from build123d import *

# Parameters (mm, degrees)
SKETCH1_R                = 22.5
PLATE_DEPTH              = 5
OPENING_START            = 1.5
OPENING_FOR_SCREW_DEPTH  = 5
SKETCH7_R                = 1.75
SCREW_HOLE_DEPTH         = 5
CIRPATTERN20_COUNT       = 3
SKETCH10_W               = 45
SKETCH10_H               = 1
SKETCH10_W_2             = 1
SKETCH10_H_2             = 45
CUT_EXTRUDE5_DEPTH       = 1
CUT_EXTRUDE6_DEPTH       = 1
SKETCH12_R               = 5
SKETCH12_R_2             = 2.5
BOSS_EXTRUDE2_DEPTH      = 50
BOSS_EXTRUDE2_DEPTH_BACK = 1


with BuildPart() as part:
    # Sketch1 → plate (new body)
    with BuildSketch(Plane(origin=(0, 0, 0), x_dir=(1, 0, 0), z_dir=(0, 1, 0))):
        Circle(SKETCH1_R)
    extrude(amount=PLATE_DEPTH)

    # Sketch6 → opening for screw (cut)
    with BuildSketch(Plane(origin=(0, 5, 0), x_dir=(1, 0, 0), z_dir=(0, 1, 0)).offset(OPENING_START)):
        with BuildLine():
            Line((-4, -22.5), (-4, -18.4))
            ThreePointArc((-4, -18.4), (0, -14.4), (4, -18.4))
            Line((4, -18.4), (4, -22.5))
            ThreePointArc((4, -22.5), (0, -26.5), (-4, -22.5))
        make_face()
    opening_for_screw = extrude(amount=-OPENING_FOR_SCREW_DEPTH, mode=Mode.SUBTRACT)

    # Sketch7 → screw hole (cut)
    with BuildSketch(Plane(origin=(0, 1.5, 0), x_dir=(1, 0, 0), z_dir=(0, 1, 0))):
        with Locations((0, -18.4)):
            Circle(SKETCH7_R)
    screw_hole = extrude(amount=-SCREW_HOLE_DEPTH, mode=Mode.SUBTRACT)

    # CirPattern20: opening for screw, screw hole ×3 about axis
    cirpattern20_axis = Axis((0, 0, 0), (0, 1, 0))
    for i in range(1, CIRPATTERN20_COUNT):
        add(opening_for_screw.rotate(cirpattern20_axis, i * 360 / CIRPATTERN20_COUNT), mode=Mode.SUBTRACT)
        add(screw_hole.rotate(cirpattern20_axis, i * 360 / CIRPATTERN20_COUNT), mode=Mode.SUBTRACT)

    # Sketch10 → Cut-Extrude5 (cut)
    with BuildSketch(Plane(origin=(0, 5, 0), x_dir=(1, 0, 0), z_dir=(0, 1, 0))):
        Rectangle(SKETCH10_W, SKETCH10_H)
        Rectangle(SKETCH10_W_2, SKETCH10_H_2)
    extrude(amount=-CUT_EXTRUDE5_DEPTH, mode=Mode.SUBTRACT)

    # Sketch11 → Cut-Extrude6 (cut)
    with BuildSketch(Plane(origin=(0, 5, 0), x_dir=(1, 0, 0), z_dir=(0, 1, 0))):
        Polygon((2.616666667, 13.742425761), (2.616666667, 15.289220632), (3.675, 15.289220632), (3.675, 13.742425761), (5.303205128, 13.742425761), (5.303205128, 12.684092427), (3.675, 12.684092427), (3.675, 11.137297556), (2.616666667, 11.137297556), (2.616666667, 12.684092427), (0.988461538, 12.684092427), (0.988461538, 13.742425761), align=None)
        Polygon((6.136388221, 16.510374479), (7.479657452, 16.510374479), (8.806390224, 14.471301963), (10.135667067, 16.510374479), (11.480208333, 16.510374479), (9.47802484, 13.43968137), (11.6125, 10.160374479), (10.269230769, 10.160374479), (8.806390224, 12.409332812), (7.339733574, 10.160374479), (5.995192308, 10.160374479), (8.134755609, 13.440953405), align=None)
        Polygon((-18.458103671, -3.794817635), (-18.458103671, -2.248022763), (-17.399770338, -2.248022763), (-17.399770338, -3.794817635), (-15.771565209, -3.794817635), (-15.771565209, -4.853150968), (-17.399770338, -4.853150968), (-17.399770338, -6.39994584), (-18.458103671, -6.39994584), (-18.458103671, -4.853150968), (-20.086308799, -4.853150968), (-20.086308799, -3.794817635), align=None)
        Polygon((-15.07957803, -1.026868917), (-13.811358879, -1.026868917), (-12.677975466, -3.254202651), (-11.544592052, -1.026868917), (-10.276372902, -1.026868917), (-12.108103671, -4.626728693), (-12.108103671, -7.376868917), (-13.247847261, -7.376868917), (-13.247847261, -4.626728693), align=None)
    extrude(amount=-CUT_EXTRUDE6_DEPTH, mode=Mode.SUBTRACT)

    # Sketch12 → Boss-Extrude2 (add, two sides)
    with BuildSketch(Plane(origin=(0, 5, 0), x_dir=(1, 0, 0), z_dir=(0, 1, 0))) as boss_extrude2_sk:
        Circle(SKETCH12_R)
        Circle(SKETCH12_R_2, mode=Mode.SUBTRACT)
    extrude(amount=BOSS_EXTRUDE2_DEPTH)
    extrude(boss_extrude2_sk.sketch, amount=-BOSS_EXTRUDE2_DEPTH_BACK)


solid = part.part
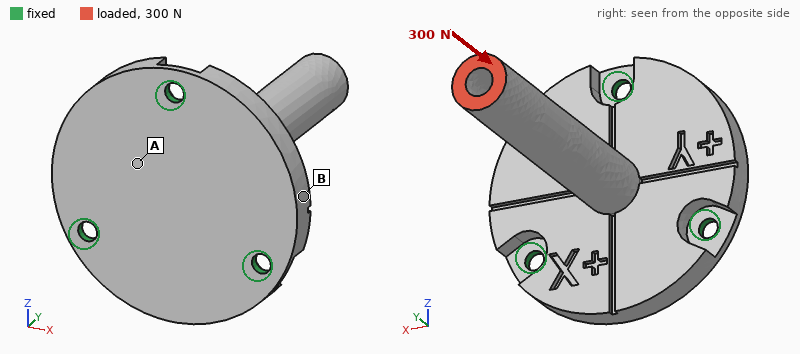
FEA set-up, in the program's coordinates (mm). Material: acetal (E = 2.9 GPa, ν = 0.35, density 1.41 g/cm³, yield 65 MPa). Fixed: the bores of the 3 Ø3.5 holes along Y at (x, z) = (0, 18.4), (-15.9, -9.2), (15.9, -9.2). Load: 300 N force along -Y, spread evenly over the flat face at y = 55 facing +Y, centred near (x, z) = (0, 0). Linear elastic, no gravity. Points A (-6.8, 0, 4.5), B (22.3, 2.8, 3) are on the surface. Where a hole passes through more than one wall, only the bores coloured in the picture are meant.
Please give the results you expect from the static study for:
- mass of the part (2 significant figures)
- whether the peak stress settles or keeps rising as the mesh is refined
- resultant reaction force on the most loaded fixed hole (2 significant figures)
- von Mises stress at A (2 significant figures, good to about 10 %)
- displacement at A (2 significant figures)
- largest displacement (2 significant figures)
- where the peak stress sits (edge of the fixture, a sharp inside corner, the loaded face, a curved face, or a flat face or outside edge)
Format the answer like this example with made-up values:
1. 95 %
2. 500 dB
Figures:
1. 14 g
2. keeps rising
3. 140 N
4. 6.0 MPa
5. 0.11 mm
6. 0.22 mm
7. edge of the fixture
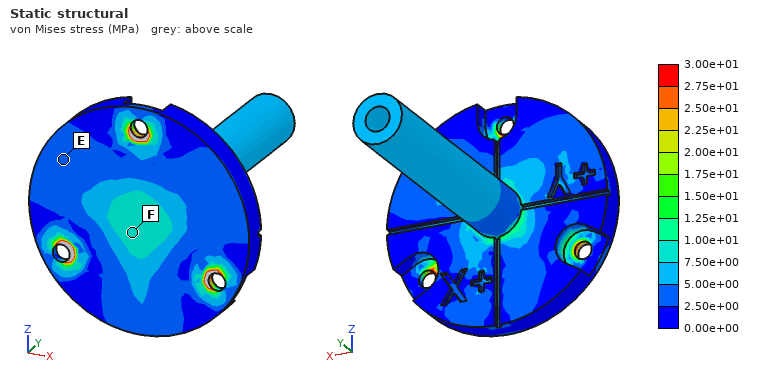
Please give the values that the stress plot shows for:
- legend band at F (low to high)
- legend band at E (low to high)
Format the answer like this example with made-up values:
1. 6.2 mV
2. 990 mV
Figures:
1. 7.50e+00 to 1.00e+01 MPa
2. 2.50e+00 to 5.00e+00 MPa
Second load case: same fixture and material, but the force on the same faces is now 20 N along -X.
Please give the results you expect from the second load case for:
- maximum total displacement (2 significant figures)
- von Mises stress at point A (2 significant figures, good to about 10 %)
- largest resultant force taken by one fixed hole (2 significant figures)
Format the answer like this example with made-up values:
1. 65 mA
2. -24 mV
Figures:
1. 0.93 mm
2. 2.5 MPa
3. 47 N
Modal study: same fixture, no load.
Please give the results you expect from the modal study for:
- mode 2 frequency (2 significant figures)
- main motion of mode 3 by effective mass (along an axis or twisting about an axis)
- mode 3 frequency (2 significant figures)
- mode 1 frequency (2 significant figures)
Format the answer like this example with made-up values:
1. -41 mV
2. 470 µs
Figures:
1. 690 Hz
2. along Y
3. 2600 Hz
4. 690 Hz
